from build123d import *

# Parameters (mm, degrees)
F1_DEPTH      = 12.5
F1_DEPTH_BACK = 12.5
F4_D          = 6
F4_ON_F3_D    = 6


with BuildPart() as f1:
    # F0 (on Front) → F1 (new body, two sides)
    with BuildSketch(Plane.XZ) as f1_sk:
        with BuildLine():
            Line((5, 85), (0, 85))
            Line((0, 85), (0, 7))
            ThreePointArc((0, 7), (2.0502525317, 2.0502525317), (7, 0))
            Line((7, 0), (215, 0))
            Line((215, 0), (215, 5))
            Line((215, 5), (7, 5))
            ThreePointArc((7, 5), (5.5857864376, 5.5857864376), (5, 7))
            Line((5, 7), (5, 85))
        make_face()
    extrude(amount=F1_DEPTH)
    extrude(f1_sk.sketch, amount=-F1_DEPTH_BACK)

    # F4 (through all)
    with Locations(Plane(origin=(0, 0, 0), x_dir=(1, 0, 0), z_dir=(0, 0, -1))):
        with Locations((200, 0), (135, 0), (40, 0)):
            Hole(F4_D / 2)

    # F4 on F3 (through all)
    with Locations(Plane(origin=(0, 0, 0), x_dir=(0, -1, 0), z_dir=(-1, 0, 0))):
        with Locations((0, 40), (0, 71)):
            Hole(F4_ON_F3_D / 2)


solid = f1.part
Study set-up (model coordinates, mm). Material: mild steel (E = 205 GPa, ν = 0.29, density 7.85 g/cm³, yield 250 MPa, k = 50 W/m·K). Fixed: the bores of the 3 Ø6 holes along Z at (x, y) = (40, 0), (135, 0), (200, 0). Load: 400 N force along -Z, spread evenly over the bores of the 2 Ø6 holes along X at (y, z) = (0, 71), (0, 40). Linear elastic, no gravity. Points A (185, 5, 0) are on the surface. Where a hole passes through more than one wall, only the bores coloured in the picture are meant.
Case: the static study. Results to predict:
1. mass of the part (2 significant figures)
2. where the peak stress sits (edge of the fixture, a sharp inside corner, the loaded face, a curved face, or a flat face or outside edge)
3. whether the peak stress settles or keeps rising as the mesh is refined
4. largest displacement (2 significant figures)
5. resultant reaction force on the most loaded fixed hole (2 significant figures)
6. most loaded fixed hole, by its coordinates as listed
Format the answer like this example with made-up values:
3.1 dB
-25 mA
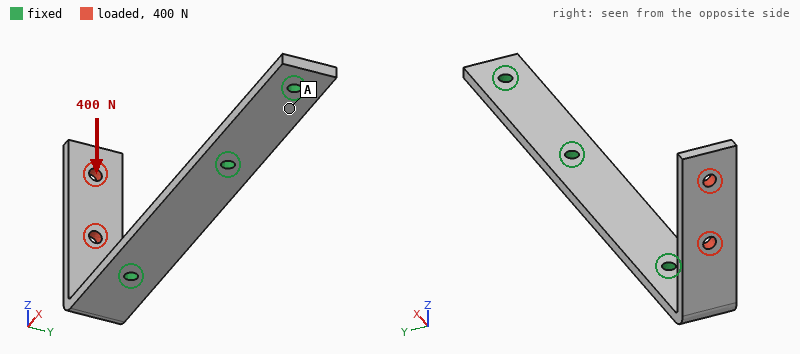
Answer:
280 g
edge of the fixture
keeps rising
0.43 mm
410 N
(40, 0)
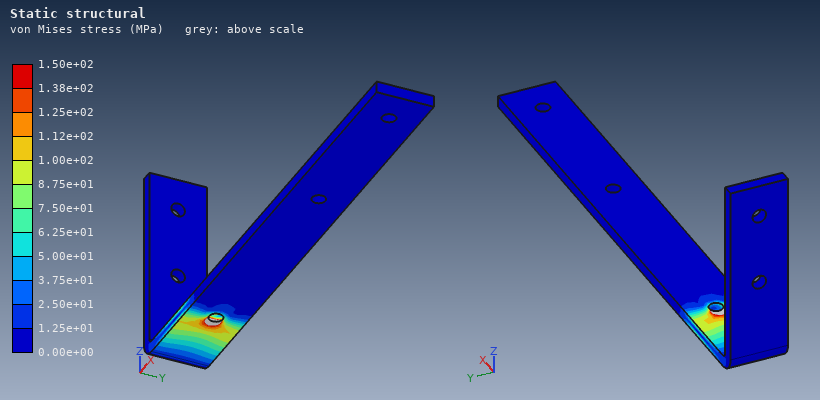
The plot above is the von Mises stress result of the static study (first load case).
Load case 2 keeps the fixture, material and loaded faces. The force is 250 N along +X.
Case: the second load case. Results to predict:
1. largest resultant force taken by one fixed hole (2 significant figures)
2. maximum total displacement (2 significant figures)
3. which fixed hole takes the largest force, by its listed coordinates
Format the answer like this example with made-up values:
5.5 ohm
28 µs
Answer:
240 N
1.2 mm
(40, 0)
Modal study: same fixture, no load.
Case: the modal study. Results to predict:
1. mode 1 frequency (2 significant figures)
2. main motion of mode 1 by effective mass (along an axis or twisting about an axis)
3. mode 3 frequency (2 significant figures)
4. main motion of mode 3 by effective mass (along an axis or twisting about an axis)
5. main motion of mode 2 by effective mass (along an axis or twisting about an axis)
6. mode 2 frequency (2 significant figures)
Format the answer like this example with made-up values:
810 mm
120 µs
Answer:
360 Hz
along X
1400 Hz
along Z
along Y
550 Hz
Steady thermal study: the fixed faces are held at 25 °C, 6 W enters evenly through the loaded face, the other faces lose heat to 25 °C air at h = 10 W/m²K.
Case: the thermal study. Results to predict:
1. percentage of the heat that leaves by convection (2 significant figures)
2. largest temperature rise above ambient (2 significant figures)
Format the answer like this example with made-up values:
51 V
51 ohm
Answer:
41 %
58 K
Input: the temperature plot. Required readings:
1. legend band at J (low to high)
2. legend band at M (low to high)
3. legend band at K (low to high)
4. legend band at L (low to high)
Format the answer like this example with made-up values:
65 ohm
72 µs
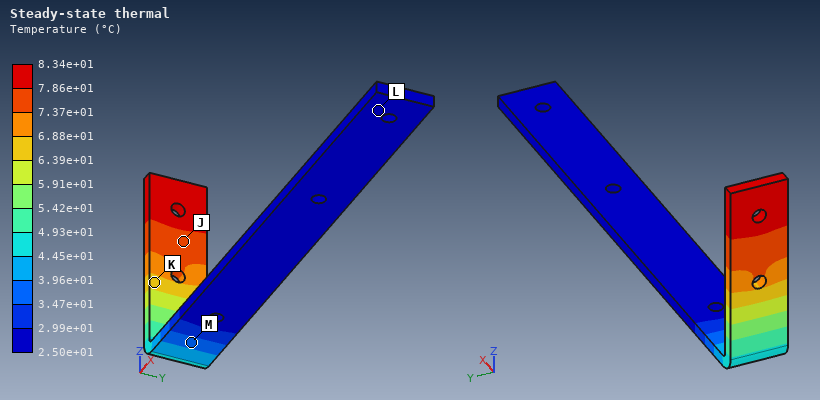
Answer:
7.37e+01 to 7.86e+01 °C
3.47e+01 to 3.96e+01 °C
6.39e+01 to 6.88e+01 °C
2.50e+01 to 2.99e+01 °C
